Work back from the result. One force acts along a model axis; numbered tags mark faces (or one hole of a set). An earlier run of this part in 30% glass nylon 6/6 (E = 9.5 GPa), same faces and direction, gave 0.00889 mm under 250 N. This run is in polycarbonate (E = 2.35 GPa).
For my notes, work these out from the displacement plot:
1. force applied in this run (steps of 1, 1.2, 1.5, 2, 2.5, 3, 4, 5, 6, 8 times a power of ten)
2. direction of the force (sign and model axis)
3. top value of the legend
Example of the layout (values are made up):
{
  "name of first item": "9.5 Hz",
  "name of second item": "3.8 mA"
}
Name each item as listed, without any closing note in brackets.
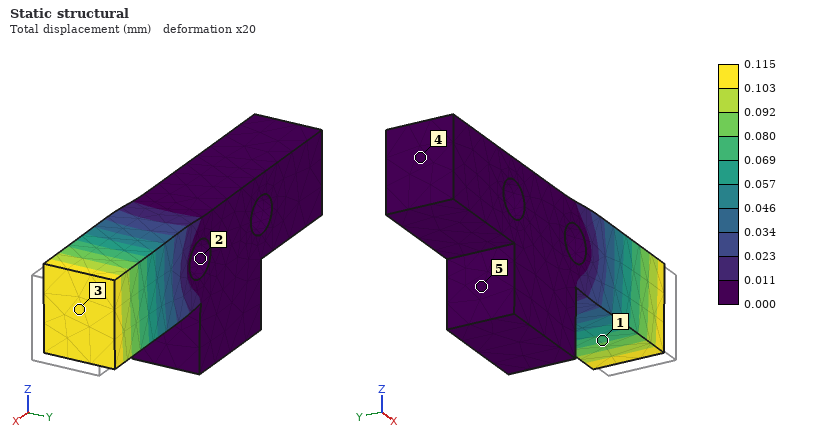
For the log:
{
  "force applied in this run": "800 N",
  "direction of the force": "-X",
  "top value of the legend": "0.115 mm"
}
